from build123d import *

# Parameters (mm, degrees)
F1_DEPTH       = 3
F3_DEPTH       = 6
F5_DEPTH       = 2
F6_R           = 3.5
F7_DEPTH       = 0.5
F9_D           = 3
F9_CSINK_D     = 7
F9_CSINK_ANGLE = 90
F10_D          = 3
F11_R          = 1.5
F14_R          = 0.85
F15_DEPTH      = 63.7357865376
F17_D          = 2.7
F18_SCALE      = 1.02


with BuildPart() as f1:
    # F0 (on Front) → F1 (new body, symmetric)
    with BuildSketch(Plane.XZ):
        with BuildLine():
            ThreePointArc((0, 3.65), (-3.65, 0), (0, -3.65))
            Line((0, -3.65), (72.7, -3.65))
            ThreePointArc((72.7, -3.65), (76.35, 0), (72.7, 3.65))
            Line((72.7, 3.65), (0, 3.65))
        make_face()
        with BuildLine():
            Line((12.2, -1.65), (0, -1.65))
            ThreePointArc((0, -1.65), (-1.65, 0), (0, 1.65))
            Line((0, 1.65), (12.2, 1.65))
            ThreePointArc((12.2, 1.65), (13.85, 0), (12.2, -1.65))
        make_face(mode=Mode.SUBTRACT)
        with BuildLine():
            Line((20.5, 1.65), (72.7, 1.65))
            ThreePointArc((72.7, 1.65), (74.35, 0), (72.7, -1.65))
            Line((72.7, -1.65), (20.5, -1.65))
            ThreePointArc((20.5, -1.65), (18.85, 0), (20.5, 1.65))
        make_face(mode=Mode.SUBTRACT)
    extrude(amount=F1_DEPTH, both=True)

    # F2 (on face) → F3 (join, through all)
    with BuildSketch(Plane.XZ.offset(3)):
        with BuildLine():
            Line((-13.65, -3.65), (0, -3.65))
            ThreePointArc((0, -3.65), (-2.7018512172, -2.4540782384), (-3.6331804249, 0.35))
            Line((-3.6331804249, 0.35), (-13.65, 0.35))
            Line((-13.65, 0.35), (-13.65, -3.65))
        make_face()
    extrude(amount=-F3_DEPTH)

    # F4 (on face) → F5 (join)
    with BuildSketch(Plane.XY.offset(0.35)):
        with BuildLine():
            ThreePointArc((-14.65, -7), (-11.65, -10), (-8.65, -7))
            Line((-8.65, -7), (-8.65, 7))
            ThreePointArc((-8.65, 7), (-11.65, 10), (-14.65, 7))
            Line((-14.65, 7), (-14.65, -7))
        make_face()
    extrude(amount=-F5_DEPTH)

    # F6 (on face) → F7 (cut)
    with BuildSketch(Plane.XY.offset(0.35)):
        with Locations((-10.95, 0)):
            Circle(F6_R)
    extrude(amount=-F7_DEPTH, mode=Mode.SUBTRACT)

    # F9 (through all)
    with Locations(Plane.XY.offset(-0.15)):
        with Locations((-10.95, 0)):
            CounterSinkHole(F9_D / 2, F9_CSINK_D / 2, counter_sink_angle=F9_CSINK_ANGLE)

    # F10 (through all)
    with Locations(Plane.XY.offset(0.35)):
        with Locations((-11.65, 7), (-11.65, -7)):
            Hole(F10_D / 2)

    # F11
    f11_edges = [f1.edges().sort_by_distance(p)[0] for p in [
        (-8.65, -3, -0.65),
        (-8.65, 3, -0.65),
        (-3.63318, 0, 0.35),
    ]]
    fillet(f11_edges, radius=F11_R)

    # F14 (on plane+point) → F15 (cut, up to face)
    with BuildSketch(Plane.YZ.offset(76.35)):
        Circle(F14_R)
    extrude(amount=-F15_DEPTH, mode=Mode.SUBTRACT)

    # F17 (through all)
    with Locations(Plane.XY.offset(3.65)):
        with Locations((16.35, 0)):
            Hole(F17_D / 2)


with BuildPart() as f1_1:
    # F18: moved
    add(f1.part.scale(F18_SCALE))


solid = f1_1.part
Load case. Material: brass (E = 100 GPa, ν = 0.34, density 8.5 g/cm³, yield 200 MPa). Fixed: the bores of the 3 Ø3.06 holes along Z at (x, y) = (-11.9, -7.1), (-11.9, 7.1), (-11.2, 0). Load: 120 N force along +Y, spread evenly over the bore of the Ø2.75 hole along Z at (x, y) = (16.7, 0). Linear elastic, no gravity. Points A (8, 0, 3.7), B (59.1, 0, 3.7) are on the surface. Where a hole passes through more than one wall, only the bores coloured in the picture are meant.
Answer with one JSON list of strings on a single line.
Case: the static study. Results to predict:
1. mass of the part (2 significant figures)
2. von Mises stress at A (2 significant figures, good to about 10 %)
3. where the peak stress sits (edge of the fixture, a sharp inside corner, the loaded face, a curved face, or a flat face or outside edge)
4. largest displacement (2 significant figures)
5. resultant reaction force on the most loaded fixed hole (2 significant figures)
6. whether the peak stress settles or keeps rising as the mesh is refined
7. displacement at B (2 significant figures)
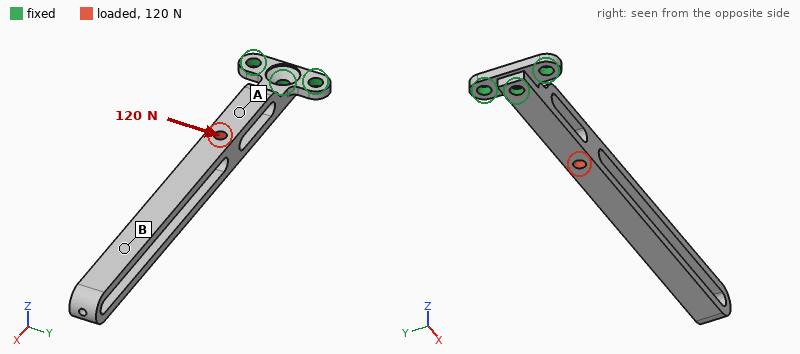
["21 g", "29 MPa", "a sharp inside corner", "0.54 mm", "250 N", "keeps rising", "0.41 mm"]
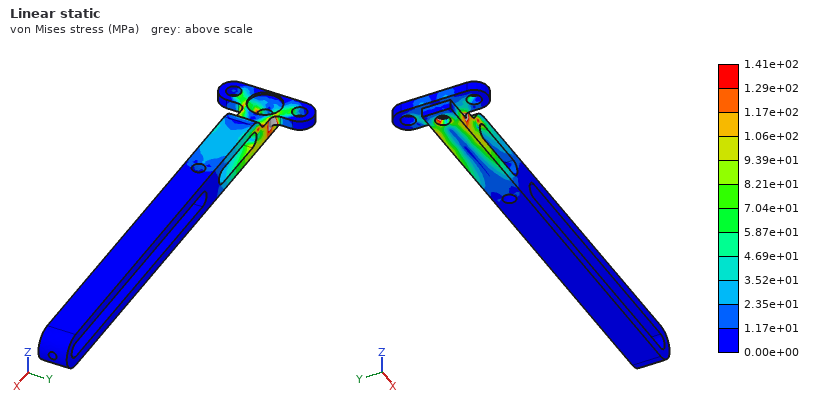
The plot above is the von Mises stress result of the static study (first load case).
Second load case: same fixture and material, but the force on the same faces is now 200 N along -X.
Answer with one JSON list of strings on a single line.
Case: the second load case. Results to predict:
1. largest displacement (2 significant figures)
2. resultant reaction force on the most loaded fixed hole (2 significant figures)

["0.14 mm", "86 N"]
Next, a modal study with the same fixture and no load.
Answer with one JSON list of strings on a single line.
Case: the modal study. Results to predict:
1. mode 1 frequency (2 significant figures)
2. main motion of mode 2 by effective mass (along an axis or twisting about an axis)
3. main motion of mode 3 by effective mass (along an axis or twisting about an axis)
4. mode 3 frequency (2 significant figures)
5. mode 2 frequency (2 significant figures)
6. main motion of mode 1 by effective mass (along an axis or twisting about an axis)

["300 Hz", "along Y", "along Z", "1500 Hz", "410 Hz", "along Z"]
